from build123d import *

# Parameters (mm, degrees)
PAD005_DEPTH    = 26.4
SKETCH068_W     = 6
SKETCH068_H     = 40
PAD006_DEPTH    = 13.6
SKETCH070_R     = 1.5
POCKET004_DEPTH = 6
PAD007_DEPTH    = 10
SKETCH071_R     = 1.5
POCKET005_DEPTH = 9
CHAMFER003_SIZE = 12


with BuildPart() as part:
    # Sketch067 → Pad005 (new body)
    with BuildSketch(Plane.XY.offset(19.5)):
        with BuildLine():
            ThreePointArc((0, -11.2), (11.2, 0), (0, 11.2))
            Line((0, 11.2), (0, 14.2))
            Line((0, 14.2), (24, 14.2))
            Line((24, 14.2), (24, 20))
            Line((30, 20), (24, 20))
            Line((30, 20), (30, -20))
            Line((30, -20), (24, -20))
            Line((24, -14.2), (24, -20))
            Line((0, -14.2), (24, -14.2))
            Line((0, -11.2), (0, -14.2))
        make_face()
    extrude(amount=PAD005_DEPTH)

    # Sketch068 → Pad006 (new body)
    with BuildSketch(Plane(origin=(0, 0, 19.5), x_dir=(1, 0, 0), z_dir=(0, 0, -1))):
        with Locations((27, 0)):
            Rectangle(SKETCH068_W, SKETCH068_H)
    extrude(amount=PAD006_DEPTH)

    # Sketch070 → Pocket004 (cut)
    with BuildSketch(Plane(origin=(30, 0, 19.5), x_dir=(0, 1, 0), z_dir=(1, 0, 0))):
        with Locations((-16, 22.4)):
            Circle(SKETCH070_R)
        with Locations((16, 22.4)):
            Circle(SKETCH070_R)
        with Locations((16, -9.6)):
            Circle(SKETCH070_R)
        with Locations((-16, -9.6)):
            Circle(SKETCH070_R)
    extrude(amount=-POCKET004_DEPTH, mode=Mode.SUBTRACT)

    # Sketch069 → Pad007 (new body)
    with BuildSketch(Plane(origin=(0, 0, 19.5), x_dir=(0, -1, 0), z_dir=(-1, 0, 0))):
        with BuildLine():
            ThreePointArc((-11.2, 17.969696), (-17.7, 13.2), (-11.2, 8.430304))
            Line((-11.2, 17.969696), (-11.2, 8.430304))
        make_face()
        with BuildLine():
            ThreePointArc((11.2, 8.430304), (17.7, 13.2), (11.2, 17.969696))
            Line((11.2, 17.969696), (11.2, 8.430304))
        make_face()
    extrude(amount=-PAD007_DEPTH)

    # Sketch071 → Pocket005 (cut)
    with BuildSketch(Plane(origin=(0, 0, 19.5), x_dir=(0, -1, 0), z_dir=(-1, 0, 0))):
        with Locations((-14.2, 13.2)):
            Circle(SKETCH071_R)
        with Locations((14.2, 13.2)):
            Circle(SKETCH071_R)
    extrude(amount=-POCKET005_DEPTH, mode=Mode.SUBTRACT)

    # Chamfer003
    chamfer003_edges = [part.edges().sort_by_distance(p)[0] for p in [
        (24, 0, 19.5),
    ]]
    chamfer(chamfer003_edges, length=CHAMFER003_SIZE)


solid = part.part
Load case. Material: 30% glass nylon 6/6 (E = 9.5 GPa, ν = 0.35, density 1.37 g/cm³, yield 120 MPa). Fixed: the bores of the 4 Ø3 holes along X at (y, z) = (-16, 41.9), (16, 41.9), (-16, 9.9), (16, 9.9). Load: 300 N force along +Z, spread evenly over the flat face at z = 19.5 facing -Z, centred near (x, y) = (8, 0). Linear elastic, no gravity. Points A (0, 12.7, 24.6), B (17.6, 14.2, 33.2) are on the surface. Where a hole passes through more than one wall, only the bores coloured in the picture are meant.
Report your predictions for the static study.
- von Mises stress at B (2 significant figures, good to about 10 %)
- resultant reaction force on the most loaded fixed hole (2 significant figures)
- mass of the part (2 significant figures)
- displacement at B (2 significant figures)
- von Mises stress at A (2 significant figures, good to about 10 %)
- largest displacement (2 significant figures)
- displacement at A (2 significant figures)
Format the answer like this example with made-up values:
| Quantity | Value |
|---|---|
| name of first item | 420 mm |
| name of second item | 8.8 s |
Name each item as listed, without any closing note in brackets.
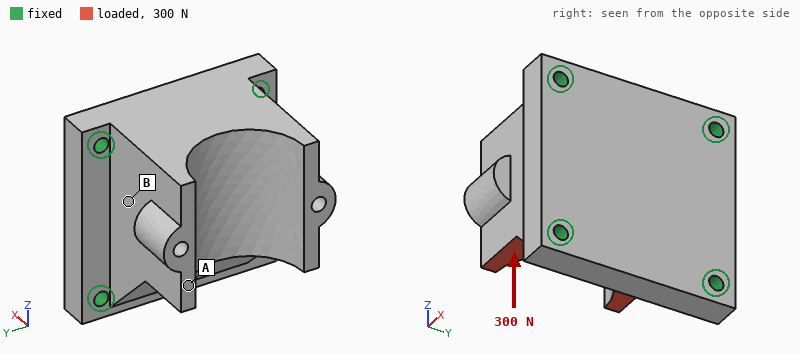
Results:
| Quantity | Value |
|---|---|
| von Mises stress at B | 1.0 MPa |
| resultant reaction force on the most loaded fixed hole | 130 N |
| mass of the part | 34 g |
| displacement at B | 3.7 µm |
| von Mises stress at A | 2.1 MPa |
| largest displacement | 13 µm |
| displacement at A | 12 µm |
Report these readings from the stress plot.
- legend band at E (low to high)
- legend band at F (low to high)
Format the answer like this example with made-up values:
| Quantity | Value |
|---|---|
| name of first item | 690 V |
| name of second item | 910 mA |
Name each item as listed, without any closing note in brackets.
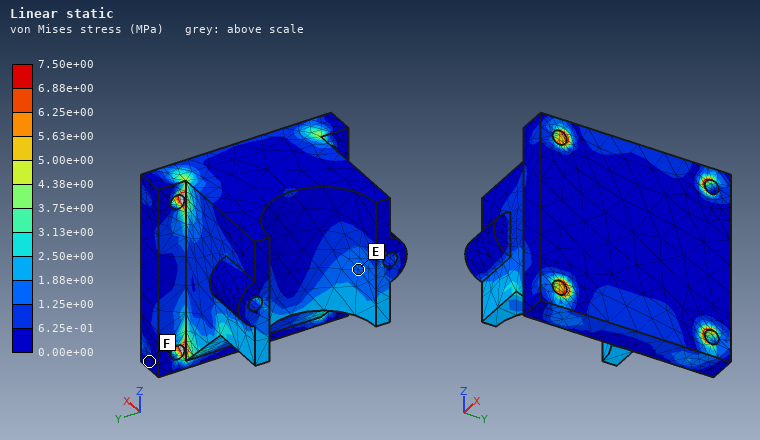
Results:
| Quantity | Value |
|---|---|
| legend band at E | 1.25e+00 to 1.88e+00 MPa |
| legend band at F | 0.00e+00 to 6.25e-01 MPa |
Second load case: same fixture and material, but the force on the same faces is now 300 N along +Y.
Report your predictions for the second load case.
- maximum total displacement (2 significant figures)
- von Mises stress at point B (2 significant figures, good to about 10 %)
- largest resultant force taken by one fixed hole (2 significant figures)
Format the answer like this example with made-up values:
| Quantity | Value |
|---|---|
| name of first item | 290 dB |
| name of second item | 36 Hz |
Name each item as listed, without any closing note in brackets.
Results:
| Quantity | Value |
|---|---|
| maximum total displacement | 39 µm |
| von Mises stress at point B | 1.9 MPa |
| largest resultant force taken by one fixed hole | 140 N |
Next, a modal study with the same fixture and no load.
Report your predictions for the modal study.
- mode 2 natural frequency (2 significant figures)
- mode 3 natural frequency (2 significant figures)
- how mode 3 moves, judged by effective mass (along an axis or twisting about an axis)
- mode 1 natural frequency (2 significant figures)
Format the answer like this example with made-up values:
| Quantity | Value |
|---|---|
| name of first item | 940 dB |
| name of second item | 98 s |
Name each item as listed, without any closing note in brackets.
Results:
| Quantity | Value |
|---|---|
| mode 2 natural frequency | 8800 Hz |
| mode 3 natural frequency | 9200 Hz |
| how mode 3 moves, judged by effective mass | along X |
| mode 1 natural frequency | 8600 Hz |
